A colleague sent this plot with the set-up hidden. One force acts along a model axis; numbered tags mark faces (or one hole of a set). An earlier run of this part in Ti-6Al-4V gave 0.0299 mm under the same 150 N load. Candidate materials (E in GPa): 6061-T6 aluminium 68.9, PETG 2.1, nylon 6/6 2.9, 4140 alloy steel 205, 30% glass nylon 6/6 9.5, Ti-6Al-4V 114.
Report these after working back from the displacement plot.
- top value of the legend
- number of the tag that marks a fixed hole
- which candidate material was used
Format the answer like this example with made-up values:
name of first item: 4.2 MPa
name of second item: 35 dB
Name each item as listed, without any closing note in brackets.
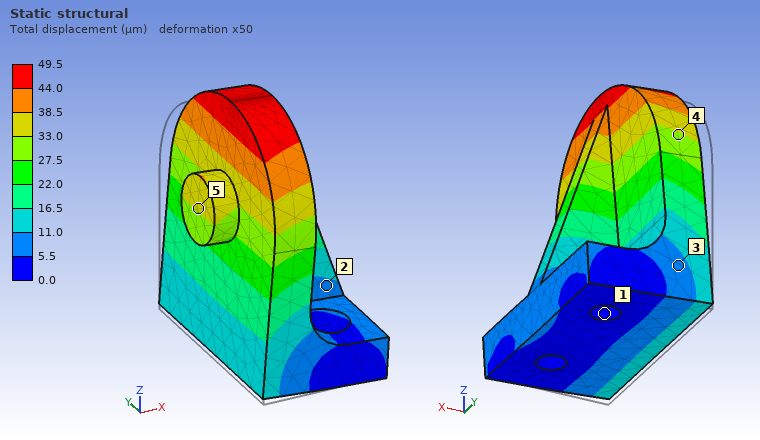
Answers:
top value of the legend: 49.5 µm
number of the tag that marks a fixed hole: 1
which candidate material was used: 6061-T6 aluminium
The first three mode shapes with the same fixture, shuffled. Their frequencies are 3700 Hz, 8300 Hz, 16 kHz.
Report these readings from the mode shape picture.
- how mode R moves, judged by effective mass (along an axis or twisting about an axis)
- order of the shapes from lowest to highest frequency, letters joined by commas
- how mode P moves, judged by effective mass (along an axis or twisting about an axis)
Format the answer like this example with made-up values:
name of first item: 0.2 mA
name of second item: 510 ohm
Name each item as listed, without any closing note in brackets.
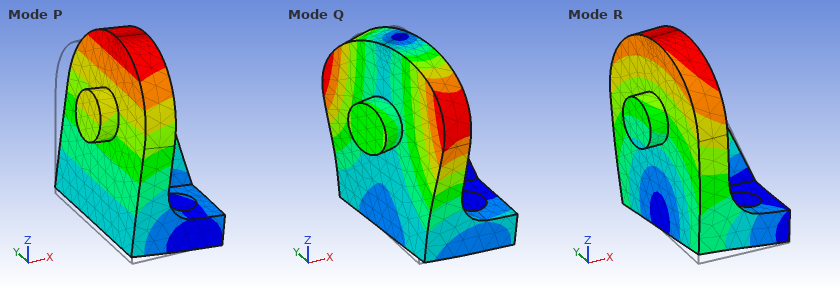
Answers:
how mode R moves, judged by effective mass: along Y
order of the shapes from lowest to highest frequency, letters joined by commas: P, R, Q
how mode P moves, judged by effective mass: along X
